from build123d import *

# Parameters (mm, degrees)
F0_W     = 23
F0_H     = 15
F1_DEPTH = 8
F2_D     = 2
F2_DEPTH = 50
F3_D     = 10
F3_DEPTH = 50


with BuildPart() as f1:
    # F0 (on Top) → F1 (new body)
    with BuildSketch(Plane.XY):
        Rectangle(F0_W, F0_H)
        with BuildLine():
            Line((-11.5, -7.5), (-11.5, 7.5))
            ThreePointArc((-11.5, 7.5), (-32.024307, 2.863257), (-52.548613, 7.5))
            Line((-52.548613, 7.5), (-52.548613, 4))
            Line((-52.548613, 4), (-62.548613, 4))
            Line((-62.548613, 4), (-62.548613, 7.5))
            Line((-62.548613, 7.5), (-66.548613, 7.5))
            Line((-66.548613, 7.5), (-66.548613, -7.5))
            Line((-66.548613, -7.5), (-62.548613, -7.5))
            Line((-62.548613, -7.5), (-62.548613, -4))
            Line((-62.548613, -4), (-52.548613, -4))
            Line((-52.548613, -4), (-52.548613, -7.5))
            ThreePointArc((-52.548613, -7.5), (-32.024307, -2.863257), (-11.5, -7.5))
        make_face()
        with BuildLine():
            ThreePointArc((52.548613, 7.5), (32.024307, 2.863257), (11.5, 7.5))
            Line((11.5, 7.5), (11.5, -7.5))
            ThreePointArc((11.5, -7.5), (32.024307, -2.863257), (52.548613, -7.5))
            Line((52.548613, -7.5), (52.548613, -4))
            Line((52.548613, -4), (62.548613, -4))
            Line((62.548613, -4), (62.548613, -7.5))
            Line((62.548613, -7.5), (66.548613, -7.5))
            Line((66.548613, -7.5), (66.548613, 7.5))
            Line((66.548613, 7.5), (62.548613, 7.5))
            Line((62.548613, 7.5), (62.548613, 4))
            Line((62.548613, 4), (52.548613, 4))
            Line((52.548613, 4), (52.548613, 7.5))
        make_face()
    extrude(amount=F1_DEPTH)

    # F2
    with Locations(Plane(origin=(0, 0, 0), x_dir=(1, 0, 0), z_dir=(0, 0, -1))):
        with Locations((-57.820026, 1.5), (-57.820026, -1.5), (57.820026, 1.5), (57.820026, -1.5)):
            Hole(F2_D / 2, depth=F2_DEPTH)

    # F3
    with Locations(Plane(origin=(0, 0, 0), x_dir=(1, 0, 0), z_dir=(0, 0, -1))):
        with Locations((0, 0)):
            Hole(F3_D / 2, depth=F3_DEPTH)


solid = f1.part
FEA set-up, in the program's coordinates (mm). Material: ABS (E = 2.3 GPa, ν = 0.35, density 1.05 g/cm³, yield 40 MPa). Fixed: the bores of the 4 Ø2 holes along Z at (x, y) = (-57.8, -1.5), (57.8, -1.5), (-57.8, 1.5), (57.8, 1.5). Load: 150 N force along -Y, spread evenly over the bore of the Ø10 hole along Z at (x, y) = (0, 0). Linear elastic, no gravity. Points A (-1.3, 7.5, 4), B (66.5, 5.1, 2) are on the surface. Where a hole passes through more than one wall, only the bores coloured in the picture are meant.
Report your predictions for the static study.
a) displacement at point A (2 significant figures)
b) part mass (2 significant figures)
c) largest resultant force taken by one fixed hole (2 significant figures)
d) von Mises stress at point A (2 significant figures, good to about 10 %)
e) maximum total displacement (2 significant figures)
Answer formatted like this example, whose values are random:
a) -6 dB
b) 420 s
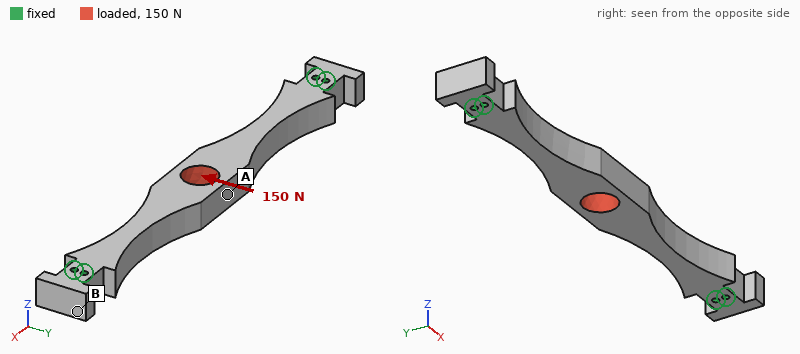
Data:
a) 0.82 mm
b) 11 g
c) 400 N
d) 9.5 MPa
e) 0.83 mm
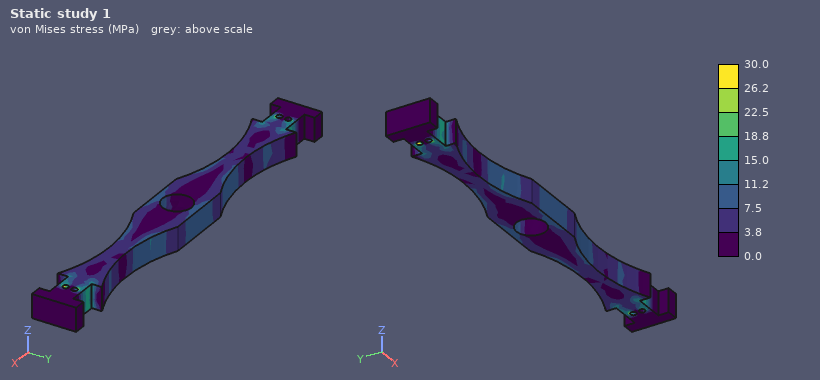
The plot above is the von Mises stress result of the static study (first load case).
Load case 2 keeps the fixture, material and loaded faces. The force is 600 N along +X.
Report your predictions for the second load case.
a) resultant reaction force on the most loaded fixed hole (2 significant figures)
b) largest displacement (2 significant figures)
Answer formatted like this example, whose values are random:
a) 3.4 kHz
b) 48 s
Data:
a) 150 N
b) 0.11 mm
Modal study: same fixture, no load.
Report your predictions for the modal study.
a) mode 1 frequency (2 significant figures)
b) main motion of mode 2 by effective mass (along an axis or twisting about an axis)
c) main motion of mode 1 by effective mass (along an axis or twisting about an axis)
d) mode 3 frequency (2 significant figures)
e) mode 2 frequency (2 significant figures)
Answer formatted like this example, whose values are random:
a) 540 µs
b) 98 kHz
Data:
a) 800 Hz
b) along Y
c) along Z
d) 2200 Hz
e) 990 Hz
